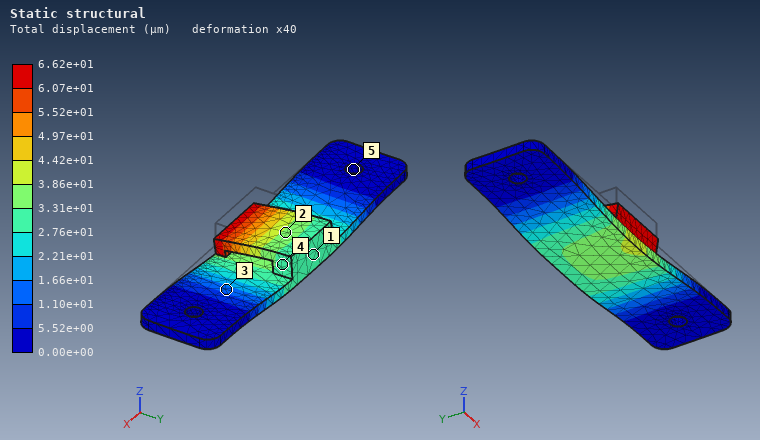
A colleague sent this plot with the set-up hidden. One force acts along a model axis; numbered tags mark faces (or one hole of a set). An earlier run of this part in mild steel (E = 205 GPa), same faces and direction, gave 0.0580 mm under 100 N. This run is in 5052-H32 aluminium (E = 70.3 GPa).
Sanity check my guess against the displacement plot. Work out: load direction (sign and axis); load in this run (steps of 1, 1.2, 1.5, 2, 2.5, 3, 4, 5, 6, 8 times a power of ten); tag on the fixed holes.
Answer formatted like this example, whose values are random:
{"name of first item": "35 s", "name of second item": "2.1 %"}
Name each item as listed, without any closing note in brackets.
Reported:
{"load direction": "-Z", "load in this run": "40 N", "tag on the fixed holes": "5"}
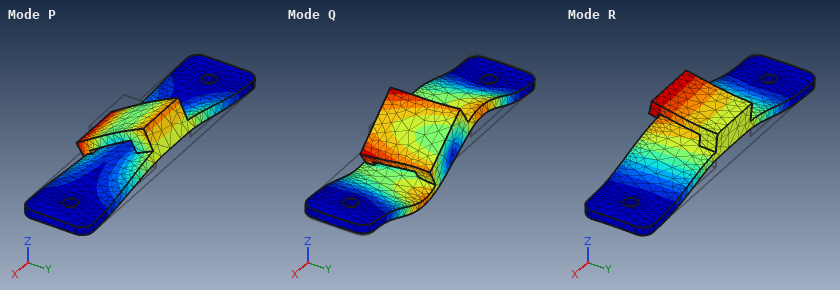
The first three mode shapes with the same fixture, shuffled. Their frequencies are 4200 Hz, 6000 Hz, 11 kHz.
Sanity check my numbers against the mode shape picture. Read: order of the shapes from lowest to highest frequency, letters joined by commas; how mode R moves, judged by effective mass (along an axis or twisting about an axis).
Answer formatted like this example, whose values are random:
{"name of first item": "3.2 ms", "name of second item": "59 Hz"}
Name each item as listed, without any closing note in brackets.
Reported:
{"order of the shapes from lowest to highest frequency, letters joined by commas": "R, P, Q", "how mode R moves, judged by effective mass": "along Z"}
